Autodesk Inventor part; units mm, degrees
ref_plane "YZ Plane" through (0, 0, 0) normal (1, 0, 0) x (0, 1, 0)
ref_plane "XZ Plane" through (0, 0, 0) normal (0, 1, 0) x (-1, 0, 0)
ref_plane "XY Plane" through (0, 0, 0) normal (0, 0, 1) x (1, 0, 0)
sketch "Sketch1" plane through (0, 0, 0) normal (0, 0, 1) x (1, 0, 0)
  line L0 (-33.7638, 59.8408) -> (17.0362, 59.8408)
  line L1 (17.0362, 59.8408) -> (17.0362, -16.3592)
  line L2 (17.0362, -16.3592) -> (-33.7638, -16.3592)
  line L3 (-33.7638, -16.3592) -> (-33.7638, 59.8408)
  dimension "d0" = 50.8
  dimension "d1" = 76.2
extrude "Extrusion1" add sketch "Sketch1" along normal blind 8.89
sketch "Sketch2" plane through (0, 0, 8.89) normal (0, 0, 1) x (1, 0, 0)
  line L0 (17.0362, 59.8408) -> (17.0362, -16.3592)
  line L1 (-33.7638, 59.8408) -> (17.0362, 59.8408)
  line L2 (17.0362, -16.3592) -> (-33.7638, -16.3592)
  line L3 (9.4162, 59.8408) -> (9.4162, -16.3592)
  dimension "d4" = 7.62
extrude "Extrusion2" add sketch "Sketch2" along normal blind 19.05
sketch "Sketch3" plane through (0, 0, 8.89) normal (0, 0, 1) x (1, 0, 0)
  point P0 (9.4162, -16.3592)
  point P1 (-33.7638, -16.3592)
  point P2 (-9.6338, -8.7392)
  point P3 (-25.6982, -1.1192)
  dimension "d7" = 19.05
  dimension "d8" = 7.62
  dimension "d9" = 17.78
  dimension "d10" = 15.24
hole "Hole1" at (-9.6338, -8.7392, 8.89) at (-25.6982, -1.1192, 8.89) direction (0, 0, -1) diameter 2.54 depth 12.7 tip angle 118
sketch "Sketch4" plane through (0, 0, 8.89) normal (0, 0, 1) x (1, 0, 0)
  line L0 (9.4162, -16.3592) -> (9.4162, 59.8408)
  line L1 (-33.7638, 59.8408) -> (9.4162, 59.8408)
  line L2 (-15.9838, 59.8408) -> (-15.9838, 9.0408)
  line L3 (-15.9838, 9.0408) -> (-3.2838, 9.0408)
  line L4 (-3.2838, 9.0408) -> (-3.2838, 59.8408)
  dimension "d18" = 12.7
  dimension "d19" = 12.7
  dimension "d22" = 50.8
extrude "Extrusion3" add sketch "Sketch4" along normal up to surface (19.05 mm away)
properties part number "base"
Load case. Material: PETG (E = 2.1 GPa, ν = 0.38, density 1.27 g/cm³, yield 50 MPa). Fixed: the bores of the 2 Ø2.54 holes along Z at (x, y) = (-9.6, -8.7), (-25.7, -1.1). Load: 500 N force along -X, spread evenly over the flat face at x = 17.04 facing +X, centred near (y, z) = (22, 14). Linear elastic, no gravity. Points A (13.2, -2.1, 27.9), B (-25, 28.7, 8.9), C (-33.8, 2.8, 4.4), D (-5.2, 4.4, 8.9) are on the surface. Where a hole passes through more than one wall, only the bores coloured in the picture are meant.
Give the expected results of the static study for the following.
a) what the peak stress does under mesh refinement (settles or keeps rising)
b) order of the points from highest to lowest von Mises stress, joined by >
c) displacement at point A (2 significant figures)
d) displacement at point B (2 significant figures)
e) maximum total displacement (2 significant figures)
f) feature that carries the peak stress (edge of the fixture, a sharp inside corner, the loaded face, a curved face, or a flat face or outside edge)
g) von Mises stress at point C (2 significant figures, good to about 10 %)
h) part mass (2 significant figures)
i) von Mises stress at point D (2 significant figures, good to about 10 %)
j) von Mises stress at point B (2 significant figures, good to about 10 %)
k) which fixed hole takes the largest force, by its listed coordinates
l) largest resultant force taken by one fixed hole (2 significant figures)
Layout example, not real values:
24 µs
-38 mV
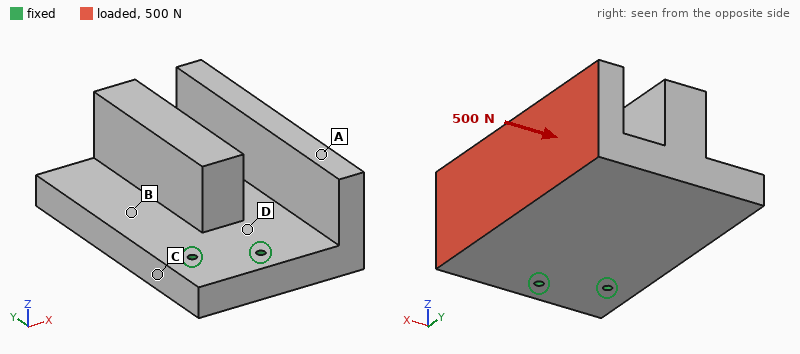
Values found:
keeps rising
D > C > B > A
0.59 mm
0.23 mm
1.1 mm
edge of the fixture
5.5 MPa
73 g
7.4 MPa
3.1 MPa
(-25.7, -1.1)
840 N
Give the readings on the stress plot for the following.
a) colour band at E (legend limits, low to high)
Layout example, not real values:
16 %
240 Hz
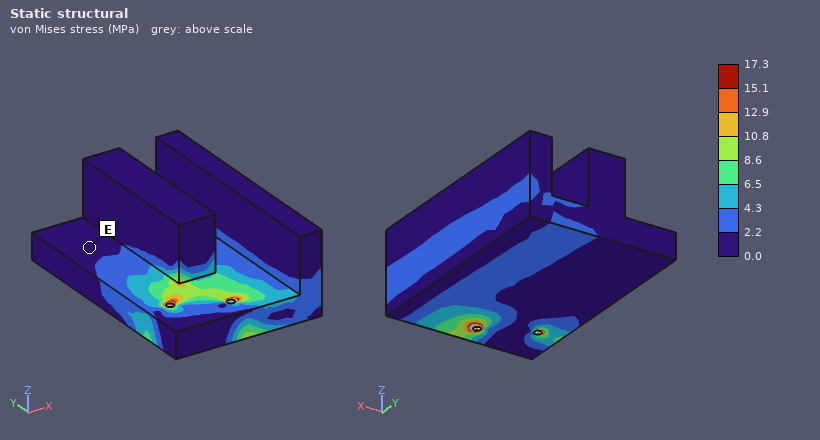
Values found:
0.0 to 2.2 MPa
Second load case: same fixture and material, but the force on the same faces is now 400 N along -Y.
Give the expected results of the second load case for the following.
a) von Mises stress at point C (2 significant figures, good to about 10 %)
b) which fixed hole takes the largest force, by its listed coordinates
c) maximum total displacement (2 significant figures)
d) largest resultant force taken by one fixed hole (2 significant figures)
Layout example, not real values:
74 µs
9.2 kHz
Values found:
4.6 MPa
(-9.6, -8.7)
1.1 mm
910 N
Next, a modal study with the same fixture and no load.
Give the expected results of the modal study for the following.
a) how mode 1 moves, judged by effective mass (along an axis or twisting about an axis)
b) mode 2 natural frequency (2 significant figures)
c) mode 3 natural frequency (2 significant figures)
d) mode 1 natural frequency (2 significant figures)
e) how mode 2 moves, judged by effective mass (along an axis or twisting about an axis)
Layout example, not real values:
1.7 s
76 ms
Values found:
along Z
650 Hz
850 Hz
270 Hz
along X
